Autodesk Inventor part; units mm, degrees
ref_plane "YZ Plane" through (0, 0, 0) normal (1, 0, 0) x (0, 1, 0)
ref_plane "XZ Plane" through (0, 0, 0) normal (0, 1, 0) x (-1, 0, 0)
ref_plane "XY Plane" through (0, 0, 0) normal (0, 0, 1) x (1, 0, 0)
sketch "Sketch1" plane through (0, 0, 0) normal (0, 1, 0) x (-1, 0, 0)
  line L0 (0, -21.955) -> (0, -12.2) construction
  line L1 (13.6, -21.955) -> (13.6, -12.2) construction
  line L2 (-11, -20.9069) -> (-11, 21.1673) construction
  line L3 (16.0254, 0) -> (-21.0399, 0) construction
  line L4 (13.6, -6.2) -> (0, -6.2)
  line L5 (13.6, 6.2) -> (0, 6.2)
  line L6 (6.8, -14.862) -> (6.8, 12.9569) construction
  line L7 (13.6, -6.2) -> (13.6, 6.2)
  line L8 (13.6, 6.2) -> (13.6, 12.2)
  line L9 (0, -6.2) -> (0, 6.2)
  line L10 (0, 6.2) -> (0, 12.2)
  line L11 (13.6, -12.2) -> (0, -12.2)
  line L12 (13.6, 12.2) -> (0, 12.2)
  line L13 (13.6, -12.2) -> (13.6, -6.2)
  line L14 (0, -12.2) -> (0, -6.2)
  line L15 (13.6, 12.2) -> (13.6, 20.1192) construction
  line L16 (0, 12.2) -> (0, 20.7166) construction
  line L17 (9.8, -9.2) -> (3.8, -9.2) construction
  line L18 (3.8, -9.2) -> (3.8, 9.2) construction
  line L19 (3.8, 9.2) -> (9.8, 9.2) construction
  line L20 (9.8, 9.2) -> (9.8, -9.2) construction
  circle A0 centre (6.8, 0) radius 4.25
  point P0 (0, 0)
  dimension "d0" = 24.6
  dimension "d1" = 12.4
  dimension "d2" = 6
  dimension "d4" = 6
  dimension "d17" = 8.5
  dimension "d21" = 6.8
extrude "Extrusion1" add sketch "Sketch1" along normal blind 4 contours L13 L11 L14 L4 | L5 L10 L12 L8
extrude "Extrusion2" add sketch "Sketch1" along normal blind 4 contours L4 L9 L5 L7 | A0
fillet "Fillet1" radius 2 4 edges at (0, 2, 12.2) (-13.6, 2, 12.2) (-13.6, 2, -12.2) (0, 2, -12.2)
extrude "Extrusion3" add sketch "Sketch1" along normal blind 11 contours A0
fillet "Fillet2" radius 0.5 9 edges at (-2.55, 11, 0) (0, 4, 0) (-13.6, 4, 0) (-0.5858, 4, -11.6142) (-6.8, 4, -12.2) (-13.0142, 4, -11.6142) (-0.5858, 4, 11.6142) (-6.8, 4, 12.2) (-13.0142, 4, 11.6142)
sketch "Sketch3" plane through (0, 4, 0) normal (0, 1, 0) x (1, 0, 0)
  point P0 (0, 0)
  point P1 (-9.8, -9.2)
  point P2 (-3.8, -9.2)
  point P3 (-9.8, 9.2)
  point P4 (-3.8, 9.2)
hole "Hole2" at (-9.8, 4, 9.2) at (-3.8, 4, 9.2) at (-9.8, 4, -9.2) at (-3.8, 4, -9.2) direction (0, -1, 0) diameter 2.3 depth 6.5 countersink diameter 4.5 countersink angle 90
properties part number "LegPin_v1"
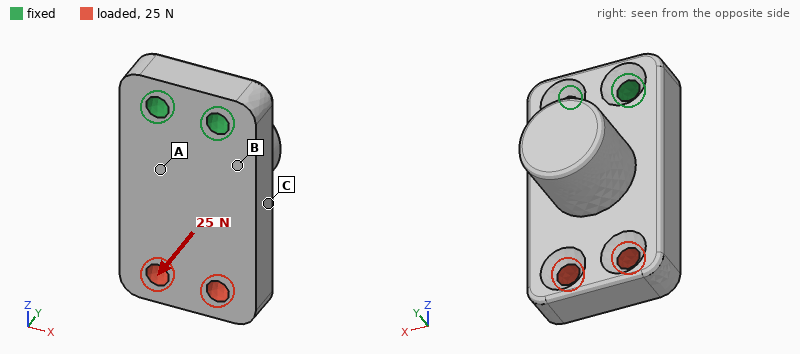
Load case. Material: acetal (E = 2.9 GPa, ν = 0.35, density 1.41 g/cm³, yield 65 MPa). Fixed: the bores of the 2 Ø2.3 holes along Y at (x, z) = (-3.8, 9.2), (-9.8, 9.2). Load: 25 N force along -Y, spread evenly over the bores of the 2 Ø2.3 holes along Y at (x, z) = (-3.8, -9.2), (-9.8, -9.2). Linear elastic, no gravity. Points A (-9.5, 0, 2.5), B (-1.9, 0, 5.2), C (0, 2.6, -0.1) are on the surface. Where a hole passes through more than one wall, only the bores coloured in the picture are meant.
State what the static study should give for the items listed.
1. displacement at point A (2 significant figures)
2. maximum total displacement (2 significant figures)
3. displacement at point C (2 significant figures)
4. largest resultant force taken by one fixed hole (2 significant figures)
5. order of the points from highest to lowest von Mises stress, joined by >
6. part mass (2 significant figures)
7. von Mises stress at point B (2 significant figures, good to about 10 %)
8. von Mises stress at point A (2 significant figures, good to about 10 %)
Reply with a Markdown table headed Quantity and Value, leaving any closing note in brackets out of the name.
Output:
| Quantity | Value |
|---|---|
| displacement at point A | 0.064 mm |
| maximum total displacement | 0.32 mm |
| displacement at point C | 0.093 mm |
| largest resultant force taken by one fixed hole | 13 N |
| order of the points from highest to lowest von Mises stress, joined by > | B > A > C |
| part mass | 2.3 g |
| von Mises stress at point B | 9.2 MPa |
| von Mises stress at point A | 6.3 MPa |
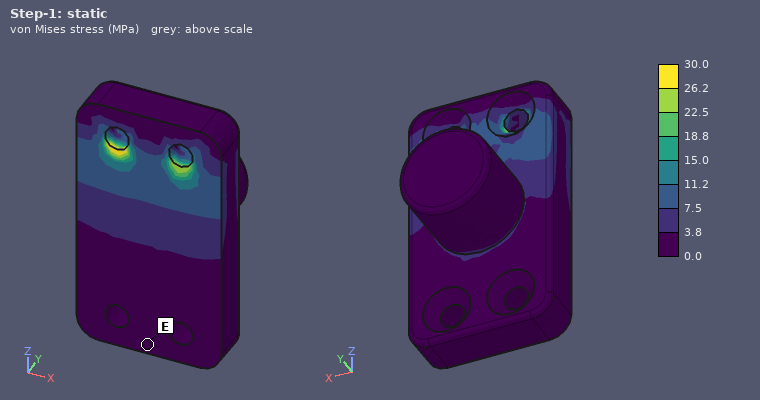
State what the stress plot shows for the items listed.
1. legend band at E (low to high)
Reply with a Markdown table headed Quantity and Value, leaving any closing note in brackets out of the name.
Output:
| Quantity | Value |
|---|---|
| legend band at E | 0.0 to 3.8 MPa |
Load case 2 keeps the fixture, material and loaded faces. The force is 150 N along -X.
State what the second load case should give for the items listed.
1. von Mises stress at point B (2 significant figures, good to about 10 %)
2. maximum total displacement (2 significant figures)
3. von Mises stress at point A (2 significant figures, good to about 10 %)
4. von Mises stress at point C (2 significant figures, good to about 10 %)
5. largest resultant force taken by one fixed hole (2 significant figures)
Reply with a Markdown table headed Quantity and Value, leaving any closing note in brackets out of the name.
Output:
| Quantity | Value |
|---|---|
| von Mises stress at point B | 14 MPa |
| maximum total displacement | 0.31 mm |
| von Mises stress at point A | 12 MPa |
| von Mises stress at point C | 11 MPa |
| largest resultant force taken by one fixed hole | 360 N |
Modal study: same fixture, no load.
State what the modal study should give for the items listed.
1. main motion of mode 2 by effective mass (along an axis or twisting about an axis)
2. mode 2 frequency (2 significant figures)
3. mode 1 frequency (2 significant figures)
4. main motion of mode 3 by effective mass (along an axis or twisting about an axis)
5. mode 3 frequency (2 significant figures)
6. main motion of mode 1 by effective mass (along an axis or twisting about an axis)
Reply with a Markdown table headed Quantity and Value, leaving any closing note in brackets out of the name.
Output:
| Quantity | Value |
|---|---|
| main motion of mode 2 by effective mass | along X |
| mode 2 frequency | 4500 Hz |
| mode 1 frequency | 1800 Hz |
| main motion of mode 3 by effective mass | twisting about Z |
| mode 3 frequency | 5300 Hz |
| main motion of mode 1 by effective mass | along Y |
